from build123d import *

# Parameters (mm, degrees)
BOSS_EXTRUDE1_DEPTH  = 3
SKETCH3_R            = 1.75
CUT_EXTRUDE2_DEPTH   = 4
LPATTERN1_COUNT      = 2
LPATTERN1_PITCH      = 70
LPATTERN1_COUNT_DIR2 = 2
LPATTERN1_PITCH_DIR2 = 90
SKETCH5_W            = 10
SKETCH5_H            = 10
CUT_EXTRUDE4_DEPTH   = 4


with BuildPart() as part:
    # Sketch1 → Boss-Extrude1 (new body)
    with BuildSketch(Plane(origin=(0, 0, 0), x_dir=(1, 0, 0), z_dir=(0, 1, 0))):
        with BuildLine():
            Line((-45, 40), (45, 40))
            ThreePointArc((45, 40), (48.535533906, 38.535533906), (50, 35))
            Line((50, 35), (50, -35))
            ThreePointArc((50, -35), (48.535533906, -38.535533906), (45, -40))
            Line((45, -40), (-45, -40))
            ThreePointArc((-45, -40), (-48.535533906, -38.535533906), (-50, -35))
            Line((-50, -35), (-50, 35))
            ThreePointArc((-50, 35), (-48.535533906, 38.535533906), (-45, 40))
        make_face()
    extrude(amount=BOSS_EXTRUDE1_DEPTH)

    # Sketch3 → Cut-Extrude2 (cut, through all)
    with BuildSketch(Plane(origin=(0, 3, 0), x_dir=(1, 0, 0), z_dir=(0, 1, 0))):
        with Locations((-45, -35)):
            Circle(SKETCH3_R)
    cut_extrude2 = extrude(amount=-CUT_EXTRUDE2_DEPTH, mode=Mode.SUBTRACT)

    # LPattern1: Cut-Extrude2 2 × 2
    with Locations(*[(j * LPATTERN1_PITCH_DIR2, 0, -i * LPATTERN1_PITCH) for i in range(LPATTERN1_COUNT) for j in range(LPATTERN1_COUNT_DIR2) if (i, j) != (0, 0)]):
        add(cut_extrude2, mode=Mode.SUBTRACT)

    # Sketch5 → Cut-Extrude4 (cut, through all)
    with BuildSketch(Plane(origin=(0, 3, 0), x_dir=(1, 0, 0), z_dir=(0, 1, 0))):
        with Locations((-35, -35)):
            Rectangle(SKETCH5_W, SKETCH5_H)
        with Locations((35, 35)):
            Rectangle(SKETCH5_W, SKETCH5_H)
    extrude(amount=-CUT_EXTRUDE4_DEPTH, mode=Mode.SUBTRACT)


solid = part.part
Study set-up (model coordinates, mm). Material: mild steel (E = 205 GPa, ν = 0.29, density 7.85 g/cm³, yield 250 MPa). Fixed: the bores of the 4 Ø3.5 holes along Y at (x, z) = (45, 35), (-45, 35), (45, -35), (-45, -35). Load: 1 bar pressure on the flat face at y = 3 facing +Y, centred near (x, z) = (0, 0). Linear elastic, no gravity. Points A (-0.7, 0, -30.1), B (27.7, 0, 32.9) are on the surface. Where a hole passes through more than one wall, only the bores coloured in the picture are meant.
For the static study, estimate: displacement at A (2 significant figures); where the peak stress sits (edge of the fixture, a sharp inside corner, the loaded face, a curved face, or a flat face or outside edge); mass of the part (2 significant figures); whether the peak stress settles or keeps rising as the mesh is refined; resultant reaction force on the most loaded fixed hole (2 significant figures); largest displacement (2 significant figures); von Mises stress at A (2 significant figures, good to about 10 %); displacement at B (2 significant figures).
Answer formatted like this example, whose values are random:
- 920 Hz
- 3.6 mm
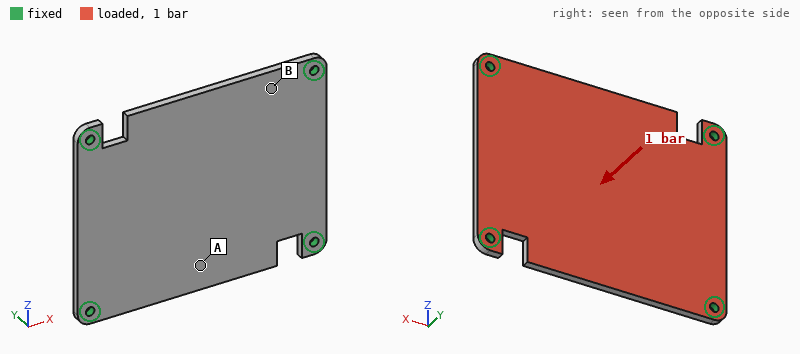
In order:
- 73 µm
- edge of the fixture
- 180 g
- keeps rising
- 210 N
- 83 µm
- 33 MPa
- 30 µm
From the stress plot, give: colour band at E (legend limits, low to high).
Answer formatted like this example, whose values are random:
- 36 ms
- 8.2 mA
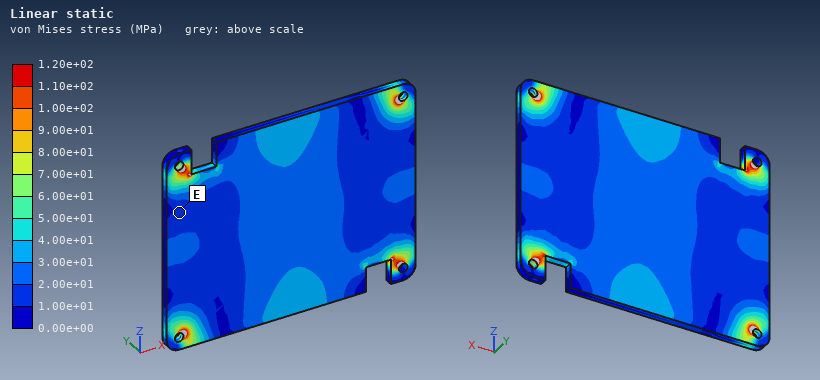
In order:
- 1.00e+01 to 2.00e+01 MPa
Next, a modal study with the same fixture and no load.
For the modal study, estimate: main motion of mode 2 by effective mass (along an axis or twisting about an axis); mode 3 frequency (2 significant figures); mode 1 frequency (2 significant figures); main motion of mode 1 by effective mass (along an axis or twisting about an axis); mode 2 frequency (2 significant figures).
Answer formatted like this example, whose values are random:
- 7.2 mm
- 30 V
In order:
- twisting about X
- 3000 Hz
- 1300 Hz
- along Y
- 2000 Hz
